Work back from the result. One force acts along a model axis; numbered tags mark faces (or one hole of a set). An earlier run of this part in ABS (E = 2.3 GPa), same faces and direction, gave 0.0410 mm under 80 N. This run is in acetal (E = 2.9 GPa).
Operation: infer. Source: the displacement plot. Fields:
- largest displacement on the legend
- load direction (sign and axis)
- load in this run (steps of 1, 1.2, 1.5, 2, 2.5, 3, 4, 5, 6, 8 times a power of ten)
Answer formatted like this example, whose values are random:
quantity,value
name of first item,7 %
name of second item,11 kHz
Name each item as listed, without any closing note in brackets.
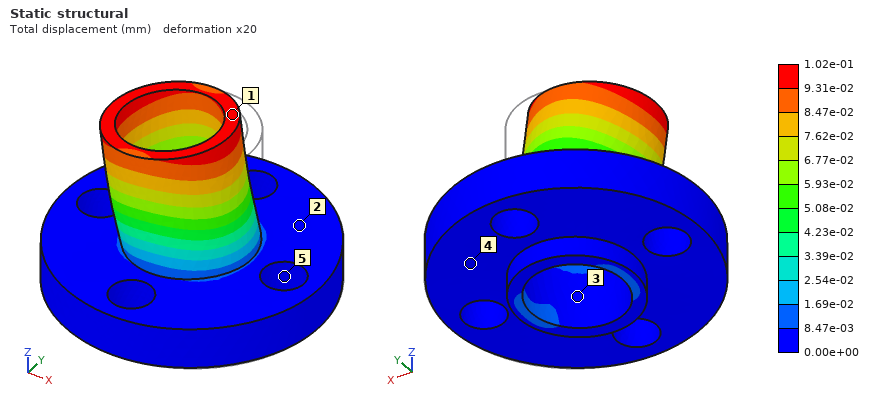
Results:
quantity,value
largest displacement on the legend,1.02e-01 mm
load direction,-X
load in this run,250 N
